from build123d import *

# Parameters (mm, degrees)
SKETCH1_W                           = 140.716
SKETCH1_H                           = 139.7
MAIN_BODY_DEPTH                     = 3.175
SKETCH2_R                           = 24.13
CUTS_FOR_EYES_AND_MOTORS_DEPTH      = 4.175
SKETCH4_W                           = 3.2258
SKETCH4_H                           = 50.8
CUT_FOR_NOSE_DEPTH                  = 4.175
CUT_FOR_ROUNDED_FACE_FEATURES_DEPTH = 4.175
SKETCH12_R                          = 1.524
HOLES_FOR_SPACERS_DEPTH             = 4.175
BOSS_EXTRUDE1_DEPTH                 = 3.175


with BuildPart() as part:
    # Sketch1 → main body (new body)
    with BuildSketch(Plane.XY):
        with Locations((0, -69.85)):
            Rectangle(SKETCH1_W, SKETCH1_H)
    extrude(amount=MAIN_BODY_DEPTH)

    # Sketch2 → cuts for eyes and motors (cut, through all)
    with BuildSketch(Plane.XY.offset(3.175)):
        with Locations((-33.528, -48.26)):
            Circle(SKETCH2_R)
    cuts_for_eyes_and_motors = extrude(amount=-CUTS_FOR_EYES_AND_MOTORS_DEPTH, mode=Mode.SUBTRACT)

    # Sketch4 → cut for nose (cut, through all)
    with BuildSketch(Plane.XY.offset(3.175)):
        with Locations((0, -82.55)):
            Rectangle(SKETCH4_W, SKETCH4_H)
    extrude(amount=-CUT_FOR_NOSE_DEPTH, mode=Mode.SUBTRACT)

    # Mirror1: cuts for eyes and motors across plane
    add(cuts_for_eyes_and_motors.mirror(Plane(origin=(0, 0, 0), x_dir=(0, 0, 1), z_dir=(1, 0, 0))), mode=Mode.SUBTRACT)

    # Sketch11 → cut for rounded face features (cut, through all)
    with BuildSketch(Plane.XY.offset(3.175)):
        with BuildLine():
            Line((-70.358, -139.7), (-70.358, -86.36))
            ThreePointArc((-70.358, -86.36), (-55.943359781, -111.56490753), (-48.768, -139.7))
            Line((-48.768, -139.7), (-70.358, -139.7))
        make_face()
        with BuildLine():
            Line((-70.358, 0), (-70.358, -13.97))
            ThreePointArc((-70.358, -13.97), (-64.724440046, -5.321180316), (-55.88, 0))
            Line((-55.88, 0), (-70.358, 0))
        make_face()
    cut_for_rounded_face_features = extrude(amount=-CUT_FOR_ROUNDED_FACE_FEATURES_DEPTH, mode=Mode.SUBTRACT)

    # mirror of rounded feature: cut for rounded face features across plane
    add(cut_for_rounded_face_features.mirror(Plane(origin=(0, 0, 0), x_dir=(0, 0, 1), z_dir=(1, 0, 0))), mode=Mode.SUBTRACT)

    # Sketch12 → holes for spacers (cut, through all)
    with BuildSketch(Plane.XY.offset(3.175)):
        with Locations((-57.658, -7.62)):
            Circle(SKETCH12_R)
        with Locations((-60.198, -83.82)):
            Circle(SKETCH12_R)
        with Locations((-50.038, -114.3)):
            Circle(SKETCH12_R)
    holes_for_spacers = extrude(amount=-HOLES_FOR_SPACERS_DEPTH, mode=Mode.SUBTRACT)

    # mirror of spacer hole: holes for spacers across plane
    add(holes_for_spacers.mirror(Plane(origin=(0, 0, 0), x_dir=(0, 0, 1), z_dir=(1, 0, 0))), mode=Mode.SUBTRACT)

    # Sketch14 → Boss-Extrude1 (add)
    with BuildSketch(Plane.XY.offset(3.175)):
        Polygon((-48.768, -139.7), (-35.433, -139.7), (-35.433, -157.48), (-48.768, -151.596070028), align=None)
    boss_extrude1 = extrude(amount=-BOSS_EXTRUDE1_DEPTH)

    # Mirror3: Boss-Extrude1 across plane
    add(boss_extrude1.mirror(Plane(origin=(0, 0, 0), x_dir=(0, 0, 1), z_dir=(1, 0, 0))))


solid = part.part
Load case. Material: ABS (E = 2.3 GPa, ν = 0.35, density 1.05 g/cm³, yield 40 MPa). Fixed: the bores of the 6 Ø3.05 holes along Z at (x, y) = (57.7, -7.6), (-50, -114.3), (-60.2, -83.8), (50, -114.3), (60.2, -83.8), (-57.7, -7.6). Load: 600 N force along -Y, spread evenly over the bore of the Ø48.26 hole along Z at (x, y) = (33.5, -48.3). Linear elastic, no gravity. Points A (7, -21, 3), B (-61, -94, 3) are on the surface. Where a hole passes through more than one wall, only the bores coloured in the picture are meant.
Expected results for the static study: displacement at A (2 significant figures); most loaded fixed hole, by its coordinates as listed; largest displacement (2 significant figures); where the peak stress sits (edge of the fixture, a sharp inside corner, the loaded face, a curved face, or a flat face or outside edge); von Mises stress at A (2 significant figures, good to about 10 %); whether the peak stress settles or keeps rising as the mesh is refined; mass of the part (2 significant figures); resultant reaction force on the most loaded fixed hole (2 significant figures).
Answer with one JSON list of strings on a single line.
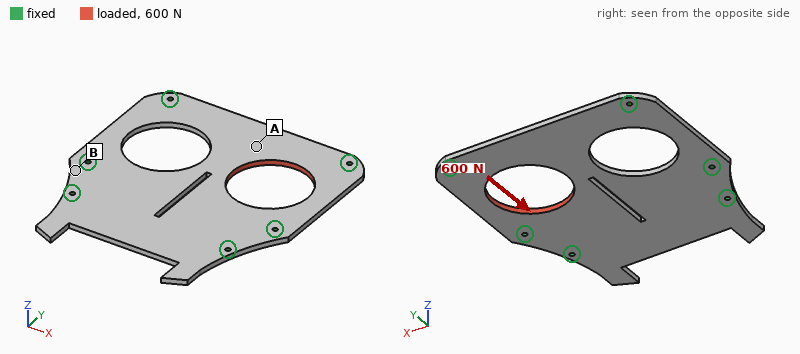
["0.089 mm", "(57.7, -7.6)", "0.10 mm", "edge of the fixture", "1.4 MPa", "keeps rising", "49 g", "190 N"]
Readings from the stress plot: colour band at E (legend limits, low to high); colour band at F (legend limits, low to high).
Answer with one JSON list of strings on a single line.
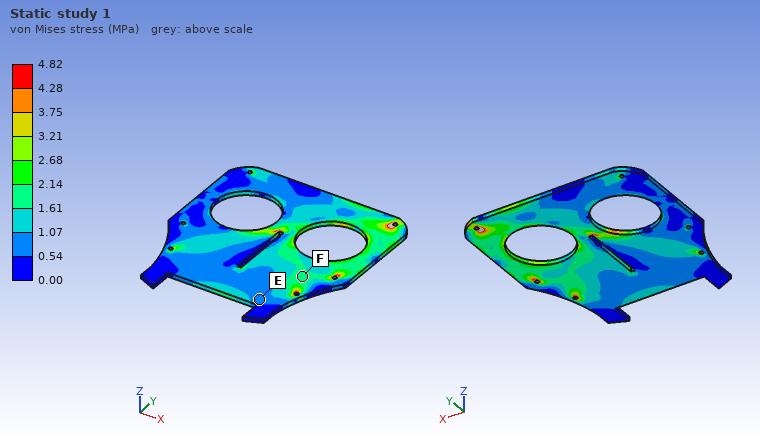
["0.54 to 1.07 MPa", "1.61 to 2.14 MPa"]
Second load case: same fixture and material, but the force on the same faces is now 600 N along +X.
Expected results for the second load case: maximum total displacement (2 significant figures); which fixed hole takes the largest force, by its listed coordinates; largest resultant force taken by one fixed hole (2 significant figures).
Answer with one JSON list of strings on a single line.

["0.13 mm", "(60.2, -83.8)", "230 N"]
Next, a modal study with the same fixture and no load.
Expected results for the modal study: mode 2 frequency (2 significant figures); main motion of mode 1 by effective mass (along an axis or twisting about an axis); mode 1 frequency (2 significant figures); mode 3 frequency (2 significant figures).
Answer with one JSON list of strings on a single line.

["370 Hz", "along Z", "290 Hz", "450 Hz"]
